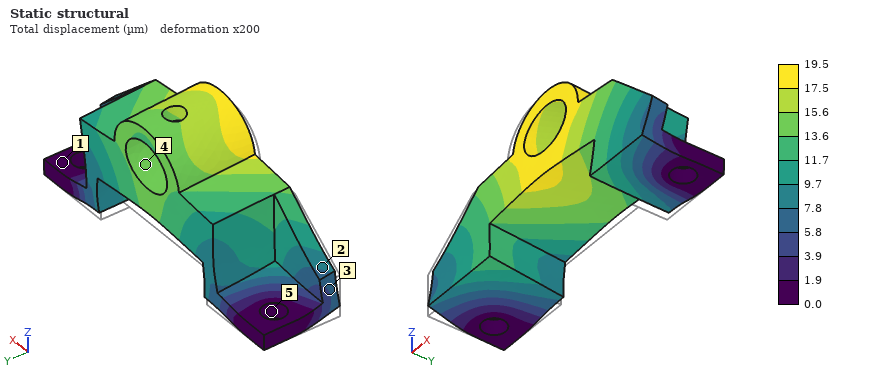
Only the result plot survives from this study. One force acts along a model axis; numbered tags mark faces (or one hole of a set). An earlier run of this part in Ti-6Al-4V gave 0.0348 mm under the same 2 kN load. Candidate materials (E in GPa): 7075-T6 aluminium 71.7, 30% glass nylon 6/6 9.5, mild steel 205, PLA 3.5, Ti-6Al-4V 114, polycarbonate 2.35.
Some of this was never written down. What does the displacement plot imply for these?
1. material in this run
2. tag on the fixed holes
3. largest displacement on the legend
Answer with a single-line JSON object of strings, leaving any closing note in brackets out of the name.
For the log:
{"material in this run": "mild steel", "tag on the fixed holes": "5", "largest displacement on the legend": "19.5 µm"}
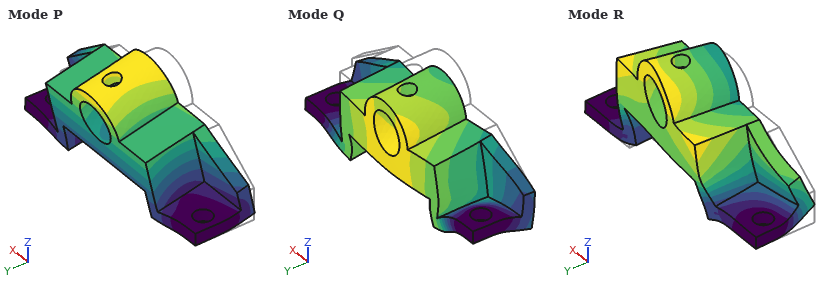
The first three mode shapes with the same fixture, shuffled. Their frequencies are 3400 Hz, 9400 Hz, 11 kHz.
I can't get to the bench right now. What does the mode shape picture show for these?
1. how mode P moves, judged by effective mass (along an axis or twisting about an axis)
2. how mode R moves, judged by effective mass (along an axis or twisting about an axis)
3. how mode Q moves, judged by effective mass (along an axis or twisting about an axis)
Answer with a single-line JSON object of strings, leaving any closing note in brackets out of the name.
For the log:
{"how mode P moves, judged by effective mass": "along Y", "how mode R moves, judged by effective mass": "along X", "how mode Q moves, judged by effective mass": "along Z"}
